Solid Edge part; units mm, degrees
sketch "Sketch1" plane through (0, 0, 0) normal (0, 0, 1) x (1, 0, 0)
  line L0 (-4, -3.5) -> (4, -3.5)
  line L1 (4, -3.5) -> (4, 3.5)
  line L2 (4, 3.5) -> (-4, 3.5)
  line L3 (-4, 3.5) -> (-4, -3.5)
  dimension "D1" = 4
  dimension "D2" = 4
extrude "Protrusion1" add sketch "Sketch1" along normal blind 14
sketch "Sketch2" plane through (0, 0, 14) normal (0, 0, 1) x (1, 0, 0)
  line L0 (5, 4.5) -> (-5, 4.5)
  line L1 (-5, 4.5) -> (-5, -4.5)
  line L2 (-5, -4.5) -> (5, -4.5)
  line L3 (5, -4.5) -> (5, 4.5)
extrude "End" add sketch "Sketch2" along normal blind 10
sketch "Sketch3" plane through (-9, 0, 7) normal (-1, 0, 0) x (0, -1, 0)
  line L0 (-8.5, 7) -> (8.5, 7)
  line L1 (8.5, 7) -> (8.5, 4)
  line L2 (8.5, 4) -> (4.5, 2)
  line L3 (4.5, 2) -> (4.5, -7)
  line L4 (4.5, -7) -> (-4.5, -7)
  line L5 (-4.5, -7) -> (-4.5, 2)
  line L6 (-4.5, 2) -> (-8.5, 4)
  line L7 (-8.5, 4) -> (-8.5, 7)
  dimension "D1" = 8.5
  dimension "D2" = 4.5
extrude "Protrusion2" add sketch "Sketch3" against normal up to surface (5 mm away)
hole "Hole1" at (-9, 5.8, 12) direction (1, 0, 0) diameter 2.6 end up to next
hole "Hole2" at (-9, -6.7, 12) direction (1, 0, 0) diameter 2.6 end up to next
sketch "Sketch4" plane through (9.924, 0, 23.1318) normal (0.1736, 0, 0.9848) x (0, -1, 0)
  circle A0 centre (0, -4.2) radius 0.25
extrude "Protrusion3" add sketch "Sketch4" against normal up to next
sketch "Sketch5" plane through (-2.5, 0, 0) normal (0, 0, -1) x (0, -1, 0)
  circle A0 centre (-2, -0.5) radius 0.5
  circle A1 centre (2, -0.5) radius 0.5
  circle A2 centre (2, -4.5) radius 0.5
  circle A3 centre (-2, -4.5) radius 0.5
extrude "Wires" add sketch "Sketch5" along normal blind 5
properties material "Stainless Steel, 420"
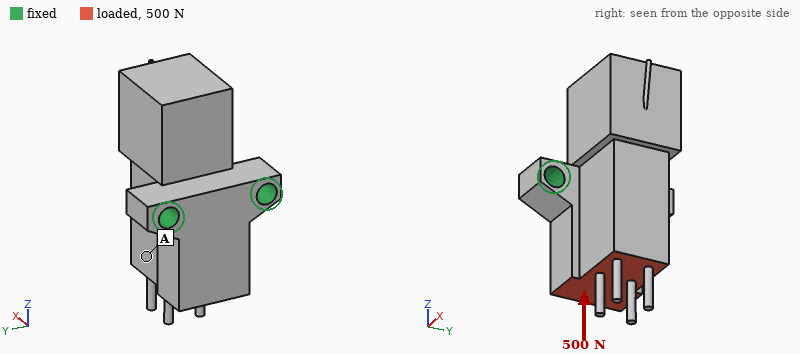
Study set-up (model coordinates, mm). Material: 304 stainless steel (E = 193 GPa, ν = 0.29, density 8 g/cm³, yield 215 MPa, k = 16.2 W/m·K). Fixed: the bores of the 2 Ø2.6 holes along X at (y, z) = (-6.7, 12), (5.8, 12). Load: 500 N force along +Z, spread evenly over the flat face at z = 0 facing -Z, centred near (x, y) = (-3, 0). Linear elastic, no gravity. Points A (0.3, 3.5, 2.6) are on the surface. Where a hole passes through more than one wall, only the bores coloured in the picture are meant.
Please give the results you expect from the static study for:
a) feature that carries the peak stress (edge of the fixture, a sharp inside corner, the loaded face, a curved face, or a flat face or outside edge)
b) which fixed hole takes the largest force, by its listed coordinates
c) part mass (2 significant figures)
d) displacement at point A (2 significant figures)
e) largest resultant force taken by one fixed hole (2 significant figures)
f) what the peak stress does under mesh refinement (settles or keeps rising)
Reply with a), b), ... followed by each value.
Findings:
a) edge of the fixture
b) (5.8, 12)
c) 20 g
d) 4.5 µm
e) 280 N
f) keeps rising
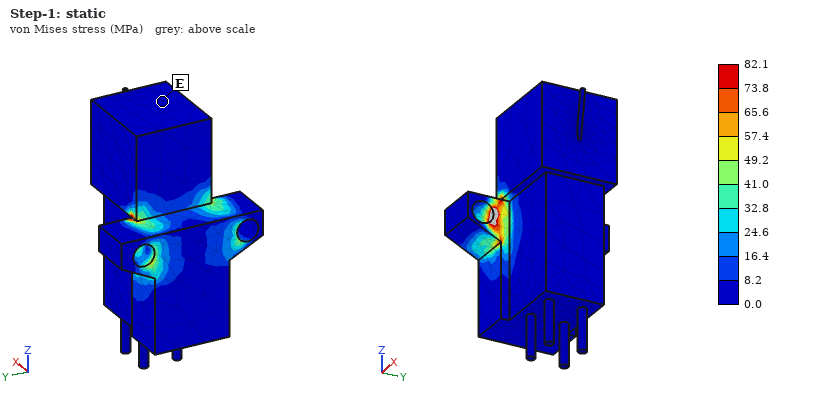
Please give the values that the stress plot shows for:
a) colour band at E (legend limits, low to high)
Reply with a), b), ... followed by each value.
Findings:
a) 0.0 to 8.2 MPa
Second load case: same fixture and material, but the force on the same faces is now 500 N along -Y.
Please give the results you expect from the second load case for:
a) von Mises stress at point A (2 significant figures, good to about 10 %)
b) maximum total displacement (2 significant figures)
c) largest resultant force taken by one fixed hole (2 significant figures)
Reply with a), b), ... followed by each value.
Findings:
a) 11 MPa
b) 8.2 µm
c) 610 N
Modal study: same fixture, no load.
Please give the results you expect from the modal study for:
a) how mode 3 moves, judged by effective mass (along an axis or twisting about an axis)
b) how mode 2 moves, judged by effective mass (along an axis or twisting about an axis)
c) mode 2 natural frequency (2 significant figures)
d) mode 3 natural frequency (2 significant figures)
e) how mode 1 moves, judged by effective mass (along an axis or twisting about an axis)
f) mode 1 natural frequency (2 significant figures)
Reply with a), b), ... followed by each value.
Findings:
a) along Y
b) along Y
c) 19 kHz
d) 22 kHz
e) along Z
f) 8400 Hz
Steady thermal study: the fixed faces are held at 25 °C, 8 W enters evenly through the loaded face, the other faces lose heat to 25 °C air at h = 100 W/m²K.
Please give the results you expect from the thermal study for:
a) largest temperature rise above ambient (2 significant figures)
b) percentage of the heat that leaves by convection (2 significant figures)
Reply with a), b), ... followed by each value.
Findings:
a) 63 K
b) 40 %
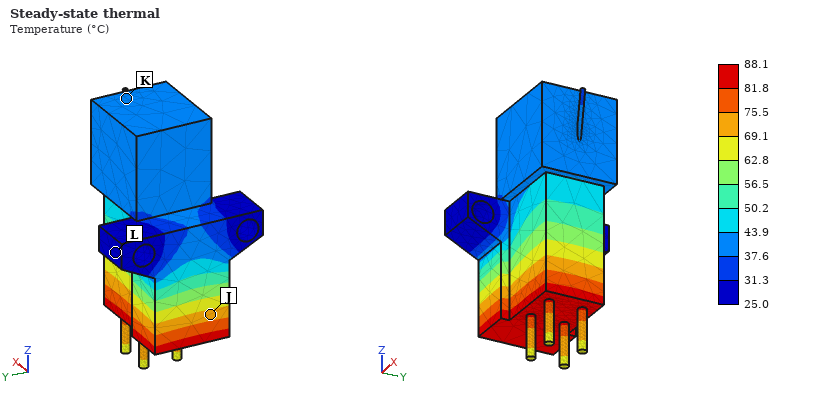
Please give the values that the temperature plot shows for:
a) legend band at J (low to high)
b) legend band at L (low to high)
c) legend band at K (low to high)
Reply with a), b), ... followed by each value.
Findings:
a) 69.1 to 75.5 °C
b) 25.0 to 31.3 °C
c) 37.6 to 43.9 °C
